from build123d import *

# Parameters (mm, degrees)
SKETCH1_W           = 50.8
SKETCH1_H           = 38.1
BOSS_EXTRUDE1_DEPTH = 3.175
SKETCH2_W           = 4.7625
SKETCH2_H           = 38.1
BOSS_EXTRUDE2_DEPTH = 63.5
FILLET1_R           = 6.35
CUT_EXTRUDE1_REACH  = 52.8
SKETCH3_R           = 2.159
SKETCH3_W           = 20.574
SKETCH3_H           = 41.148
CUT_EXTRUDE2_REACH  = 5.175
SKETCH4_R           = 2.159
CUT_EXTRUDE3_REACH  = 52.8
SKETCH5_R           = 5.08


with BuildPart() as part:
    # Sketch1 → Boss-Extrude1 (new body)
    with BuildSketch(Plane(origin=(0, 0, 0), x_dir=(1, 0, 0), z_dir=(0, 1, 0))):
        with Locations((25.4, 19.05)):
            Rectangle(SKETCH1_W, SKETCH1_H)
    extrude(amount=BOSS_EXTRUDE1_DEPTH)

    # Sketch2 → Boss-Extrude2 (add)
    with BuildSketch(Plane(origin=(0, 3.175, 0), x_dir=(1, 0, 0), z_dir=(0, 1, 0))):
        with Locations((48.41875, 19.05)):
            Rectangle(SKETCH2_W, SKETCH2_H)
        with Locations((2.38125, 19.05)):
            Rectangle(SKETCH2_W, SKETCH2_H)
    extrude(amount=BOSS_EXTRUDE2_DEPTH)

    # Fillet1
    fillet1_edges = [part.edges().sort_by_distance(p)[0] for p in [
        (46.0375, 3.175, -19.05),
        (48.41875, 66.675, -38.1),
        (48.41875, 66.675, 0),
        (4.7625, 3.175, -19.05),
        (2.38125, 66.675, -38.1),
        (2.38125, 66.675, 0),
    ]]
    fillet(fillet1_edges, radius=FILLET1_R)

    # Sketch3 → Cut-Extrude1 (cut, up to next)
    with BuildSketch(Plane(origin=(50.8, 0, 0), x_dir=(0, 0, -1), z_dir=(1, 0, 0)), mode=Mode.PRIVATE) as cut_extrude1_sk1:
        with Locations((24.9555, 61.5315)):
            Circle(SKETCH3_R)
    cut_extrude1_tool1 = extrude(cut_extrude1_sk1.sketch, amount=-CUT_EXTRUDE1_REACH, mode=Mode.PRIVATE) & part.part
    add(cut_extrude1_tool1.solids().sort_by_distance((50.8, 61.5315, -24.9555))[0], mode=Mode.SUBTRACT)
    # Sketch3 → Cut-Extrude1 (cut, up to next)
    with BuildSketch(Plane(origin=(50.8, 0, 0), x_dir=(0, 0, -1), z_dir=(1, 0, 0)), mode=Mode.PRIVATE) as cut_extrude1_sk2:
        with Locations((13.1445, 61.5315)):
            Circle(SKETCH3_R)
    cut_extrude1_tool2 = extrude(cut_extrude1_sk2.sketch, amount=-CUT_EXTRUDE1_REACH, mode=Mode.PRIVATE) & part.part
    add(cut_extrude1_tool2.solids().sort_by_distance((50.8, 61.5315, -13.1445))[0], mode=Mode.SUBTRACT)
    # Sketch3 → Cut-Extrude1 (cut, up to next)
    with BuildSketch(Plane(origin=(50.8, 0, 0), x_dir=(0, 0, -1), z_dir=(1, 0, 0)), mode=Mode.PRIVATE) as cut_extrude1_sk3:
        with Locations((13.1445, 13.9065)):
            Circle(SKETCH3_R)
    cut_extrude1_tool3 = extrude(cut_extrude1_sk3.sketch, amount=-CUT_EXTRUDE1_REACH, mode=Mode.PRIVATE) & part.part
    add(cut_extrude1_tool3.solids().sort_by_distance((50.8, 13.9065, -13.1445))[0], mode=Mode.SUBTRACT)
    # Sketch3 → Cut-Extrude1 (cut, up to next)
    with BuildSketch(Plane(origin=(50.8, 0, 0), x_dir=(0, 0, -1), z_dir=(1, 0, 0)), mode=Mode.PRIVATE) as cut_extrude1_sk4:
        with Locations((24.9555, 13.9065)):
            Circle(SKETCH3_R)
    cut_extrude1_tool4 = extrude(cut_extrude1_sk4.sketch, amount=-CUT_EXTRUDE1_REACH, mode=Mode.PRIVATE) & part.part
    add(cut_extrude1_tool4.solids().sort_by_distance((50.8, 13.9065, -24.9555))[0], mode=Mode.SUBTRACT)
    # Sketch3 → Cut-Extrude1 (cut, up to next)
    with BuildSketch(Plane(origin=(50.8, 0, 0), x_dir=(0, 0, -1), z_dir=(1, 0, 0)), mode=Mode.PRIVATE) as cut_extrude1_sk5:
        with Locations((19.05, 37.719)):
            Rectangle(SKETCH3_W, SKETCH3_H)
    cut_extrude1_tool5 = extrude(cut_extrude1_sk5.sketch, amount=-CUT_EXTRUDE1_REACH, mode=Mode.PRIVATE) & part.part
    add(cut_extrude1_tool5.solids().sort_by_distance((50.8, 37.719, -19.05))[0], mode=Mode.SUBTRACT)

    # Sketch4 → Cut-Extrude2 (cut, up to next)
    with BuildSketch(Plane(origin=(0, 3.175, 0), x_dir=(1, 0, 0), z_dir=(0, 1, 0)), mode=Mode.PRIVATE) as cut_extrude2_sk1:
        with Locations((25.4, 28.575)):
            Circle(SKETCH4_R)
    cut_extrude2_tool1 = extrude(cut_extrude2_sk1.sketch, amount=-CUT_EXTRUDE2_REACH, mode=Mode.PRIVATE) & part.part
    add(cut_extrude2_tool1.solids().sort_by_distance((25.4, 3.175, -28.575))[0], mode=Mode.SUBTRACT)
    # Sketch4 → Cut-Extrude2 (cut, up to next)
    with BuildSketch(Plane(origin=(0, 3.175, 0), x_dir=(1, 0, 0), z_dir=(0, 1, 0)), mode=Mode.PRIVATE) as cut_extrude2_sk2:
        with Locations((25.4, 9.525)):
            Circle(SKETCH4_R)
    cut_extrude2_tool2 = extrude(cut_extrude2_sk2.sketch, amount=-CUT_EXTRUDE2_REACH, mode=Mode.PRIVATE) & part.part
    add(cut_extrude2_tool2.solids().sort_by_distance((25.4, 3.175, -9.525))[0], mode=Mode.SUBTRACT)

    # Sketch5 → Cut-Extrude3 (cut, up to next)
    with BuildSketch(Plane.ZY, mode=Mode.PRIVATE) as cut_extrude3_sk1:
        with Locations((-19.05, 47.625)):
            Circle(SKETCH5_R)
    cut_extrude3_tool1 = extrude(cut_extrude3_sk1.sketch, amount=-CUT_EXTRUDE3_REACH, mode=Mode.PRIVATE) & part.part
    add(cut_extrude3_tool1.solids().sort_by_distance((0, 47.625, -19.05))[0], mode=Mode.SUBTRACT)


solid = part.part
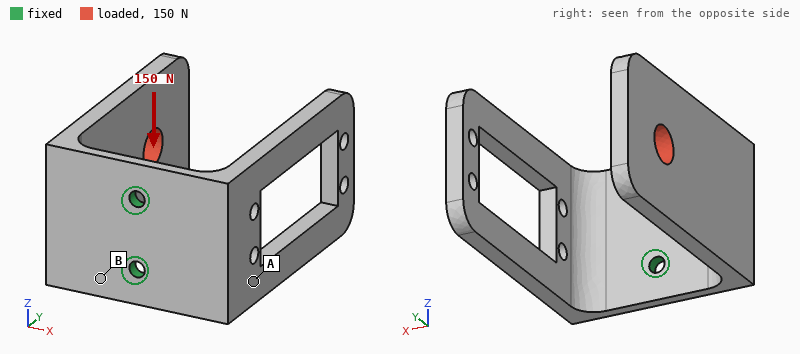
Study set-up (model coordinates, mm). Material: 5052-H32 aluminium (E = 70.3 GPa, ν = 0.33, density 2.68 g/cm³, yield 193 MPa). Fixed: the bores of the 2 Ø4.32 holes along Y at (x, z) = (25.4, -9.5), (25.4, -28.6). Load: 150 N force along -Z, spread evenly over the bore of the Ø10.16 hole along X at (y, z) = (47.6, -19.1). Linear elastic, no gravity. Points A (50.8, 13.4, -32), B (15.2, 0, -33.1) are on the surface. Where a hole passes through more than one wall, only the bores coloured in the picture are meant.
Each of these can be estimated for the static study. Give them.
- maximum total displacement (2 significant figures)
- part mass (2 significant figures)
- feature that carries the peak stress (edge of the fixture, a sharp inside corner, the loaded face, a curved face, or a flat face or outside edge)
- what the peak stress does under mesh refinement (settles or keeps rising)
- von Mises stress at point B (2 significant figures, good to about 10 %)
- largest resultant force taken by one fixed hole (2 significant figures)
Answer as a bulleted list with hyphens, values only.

- 0.30 mm
- 67 g
- edge of the fixture
- keeps rising
- 28 MPa
- 330 N
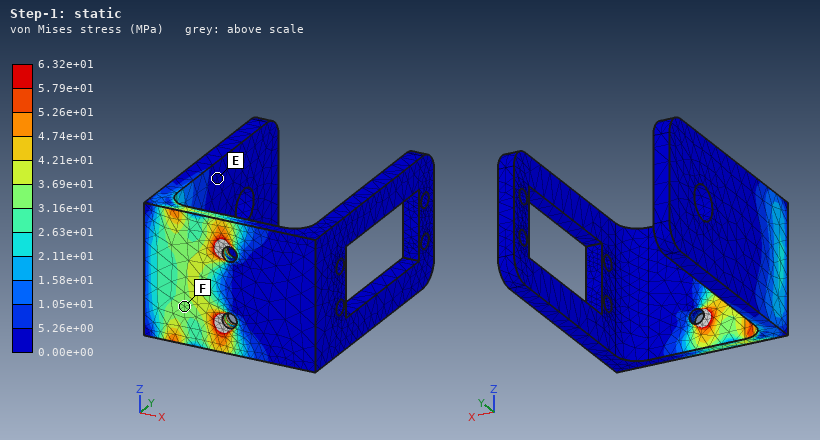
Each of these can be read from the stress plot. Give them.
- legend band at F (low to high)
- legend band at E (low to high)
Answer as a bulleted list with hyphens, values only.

- 3.16e+01 to 3.69e+01 MPa
- 0.00e+00 to 5.26e+00 MPa
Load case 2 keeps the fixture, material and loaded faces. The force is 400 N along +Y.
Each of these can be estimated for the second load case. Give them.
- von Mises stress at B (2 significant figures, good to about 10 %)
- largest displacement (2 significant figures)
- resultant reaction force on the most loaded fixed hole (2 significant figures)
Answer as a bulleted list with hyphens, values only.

- 73 MPa
- 0.86 mm
- 200 N
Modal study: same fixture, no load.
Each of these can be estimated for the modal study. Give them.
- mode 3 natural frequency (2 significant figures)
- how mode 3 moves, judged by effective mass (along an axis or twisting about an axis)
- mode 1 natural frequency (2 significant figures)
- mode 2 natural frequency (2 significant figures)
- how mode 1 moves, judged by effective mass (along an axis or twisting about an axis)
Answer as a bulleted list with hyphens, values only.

- 920 Hz
- along Z
- 440 Hz
- 520 Hz
- along X
